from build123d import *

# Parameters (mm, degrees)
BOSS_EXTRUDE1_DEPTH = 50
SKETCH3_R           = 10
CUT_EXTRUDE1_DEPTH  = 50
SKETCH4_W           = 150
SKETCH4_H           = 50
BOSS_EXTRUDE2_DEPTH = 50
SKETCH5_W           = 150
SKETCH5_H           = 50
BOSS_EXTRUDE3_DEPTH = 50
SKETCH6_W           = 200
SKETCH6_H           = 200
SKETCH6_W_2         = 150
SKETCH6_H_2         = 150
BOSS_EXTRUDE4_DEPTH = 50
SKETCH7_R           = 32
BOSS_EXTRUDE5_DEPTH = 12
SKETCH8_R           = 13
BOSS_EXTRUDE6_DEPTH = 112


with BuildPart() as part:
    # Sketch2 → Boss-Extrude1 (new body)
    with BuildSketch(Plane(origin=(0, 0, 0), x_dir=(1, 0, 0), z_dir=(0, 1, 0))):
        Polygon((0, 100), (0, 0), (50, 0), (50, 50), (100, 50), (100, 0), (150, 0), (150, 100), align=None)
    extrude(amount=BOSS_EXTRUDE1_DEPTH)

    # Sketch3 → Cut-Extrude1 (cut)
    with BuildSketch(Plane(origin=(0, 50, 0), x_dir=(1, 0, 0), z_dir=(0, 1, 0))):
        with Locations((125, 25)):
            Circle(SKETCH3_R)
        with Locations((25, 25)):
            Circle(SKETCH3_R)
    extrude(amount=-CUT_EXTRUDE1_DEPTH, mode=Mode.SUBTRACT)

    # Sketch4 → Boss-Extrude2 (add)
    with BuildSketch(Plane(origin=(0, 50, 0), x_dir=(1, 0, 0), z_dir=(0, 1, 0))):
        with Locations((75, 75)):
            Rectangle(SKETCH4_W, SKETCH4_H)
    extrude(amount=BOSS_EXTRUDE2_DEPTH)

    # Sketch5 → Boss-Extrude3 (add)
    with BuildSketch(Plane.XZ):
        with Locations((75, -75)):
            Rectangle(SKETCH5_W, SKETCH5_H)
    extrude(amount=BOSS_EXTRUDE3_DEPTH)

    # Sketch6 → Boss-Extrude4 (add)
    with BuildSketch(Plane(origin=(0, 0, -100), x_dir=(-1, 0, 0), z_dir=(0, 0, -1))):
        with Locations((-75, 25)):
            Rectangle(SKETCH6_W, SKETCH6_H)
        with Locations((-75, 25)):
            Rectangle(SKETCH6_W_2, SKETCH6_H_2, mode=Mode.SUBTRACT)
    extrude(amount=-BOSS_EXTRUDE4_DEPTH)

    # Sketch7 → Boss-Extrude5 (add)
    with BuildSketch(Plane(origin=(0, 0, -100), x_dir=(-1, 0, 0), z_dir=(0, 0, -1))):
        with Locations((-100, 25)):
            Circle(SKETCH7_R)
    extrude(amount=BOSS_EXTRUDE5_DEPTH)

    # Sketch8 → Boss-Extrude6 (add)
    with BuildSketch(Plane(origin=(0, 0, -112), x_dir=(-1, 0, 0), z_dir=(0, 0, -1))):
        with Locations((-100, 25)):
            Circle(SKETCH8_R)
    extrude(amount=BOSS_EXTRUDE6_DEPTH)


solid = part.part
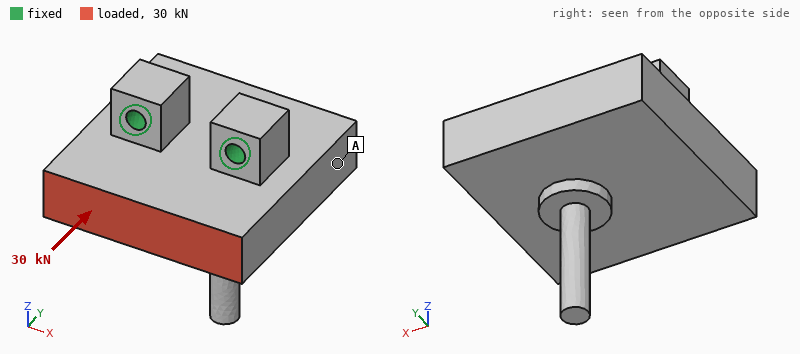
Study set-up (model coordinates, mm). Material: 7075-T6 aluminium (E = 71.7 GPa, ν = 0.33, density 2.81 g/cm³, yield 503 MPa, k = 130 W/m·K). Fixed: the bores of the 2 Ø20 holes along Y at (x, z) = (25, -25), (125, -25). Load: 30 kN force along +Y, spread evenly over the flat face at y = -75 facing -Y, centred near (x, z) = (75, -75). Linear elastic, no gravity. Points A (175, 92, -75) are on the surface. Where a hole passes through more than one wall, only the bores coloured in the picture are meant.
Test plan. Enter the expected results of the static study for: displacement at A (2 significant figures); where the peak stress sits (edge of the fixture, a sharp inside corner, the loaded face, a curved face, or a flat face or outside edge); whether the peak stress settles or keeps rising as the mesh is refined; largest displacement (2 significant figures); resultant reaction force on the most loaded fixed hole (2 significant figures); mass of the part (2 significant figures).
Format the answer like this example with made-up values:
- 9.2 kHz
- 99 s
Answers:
- 37 µm
- edge of the fixture
- keeps rising
- 87 µm
- 15 kN
- 6.5 kg
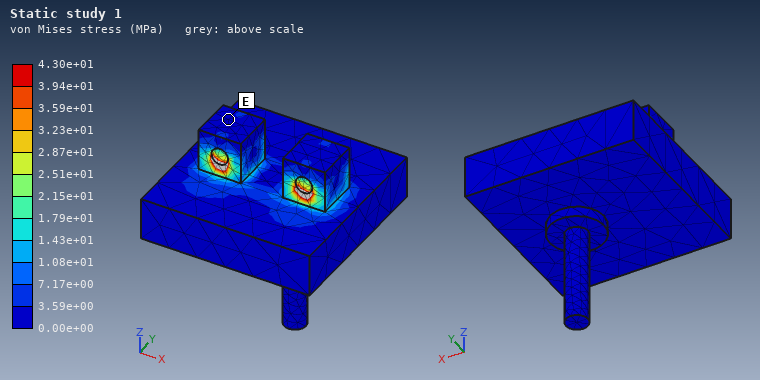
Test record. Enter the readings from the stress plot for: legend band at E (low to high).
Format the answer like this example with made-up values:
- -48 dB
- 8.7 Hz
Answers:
- 0.00e+00 to 3.59e+00 MPa
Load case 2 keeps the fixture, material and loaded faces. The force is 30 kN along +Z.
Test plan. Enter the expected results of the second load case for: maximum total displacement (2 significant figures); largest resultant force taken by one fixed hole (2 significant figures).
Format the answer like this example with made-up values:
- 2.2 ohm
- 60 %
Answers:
- 0.25 mm
- 15 kN
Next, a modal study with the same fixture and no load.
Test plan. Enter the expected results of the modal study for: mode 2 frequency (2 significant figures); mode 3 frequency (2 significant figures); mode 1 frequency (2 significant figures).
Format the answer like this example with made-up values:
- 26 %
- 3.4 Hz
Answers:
- 1300 Hz
- 1500 Hz
- 1200 Hz
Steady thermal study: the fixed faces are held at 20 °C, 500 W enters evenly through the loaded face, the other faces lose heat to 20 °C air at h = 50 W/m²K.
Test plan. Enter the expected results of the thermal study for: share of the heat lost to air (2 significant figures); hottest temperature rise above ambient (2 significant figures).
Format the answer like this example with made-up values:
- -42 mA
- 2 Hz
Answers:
- 26 %
- 50 K
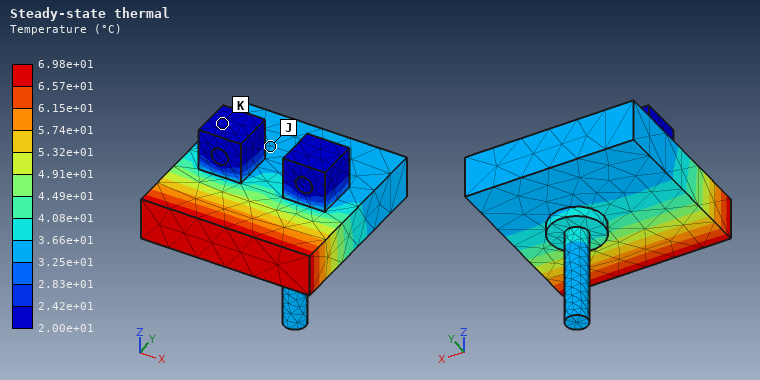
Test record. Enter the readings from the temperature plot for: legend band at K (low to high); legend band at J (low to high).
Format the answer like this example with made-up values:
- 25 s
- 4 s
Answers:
- 2.00e+01 to 2.42e+01 °C
- 3.25e+01 to 3.66e+01 °C
